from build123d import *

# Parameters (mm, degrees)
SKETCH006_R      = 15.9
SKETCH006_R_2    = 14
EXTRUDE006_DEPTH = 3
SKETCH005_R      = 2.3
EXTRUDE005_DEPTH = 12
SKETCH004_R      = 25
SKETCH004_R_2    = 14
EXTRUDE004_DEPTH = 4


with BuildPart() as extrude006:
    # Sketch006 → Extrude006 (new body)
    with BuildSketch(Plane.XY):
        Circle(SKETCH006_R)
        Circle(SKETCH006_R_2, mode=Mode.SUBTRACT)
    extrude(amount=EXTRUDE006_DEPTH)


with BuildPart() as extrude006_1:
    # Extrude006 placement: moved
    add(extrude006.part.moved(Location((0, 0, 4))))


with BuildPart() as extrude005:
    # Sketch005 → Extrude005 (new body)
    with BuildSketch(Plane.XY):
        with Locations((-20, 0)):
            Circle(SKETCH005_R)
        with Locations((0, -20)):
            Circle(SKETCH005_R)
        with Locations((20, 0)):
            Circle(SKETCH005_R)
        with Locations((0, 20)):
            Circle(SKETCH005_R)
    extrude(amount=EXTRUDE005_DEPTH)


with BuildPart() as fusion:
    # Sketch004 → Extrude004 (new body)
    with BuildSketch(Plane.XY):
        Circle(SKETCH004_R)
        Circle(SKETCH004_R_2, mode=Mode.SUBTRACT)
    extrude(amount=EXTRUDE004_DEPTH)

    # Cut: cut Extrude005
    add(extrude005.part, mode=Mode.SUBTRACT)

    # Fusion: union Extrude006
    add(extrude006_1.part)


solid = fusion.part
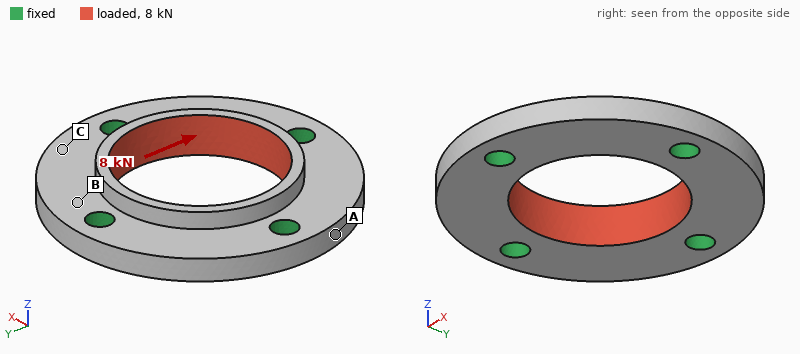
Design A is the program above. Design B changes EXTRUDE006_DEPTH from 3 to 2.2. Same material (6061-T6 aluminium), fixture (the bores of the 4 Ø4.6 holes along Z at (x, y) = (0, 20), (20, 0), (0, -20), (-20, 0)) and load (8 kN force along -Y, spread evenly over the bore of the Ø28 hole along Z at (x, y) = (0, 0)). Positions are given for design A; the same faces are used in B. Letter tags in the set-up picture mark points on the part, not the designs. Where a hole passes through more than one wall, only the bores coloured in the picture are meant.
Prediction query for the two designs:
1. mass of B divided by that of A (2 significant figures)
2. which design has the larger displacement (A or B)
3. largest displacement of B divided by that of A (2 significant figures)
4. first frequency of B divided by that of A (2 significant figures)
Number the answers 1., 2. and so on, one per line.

1. 0.97
2. A
3. 0.84
4. 1.0
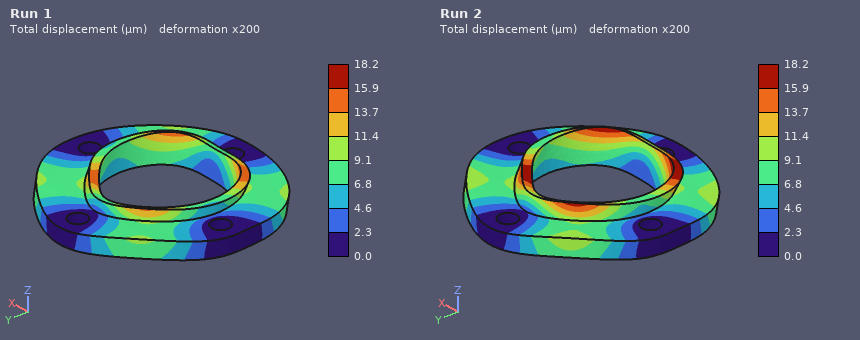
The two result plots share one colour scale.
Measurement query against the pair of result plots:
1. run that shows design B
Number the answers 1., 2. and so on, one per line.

1. Run 1
